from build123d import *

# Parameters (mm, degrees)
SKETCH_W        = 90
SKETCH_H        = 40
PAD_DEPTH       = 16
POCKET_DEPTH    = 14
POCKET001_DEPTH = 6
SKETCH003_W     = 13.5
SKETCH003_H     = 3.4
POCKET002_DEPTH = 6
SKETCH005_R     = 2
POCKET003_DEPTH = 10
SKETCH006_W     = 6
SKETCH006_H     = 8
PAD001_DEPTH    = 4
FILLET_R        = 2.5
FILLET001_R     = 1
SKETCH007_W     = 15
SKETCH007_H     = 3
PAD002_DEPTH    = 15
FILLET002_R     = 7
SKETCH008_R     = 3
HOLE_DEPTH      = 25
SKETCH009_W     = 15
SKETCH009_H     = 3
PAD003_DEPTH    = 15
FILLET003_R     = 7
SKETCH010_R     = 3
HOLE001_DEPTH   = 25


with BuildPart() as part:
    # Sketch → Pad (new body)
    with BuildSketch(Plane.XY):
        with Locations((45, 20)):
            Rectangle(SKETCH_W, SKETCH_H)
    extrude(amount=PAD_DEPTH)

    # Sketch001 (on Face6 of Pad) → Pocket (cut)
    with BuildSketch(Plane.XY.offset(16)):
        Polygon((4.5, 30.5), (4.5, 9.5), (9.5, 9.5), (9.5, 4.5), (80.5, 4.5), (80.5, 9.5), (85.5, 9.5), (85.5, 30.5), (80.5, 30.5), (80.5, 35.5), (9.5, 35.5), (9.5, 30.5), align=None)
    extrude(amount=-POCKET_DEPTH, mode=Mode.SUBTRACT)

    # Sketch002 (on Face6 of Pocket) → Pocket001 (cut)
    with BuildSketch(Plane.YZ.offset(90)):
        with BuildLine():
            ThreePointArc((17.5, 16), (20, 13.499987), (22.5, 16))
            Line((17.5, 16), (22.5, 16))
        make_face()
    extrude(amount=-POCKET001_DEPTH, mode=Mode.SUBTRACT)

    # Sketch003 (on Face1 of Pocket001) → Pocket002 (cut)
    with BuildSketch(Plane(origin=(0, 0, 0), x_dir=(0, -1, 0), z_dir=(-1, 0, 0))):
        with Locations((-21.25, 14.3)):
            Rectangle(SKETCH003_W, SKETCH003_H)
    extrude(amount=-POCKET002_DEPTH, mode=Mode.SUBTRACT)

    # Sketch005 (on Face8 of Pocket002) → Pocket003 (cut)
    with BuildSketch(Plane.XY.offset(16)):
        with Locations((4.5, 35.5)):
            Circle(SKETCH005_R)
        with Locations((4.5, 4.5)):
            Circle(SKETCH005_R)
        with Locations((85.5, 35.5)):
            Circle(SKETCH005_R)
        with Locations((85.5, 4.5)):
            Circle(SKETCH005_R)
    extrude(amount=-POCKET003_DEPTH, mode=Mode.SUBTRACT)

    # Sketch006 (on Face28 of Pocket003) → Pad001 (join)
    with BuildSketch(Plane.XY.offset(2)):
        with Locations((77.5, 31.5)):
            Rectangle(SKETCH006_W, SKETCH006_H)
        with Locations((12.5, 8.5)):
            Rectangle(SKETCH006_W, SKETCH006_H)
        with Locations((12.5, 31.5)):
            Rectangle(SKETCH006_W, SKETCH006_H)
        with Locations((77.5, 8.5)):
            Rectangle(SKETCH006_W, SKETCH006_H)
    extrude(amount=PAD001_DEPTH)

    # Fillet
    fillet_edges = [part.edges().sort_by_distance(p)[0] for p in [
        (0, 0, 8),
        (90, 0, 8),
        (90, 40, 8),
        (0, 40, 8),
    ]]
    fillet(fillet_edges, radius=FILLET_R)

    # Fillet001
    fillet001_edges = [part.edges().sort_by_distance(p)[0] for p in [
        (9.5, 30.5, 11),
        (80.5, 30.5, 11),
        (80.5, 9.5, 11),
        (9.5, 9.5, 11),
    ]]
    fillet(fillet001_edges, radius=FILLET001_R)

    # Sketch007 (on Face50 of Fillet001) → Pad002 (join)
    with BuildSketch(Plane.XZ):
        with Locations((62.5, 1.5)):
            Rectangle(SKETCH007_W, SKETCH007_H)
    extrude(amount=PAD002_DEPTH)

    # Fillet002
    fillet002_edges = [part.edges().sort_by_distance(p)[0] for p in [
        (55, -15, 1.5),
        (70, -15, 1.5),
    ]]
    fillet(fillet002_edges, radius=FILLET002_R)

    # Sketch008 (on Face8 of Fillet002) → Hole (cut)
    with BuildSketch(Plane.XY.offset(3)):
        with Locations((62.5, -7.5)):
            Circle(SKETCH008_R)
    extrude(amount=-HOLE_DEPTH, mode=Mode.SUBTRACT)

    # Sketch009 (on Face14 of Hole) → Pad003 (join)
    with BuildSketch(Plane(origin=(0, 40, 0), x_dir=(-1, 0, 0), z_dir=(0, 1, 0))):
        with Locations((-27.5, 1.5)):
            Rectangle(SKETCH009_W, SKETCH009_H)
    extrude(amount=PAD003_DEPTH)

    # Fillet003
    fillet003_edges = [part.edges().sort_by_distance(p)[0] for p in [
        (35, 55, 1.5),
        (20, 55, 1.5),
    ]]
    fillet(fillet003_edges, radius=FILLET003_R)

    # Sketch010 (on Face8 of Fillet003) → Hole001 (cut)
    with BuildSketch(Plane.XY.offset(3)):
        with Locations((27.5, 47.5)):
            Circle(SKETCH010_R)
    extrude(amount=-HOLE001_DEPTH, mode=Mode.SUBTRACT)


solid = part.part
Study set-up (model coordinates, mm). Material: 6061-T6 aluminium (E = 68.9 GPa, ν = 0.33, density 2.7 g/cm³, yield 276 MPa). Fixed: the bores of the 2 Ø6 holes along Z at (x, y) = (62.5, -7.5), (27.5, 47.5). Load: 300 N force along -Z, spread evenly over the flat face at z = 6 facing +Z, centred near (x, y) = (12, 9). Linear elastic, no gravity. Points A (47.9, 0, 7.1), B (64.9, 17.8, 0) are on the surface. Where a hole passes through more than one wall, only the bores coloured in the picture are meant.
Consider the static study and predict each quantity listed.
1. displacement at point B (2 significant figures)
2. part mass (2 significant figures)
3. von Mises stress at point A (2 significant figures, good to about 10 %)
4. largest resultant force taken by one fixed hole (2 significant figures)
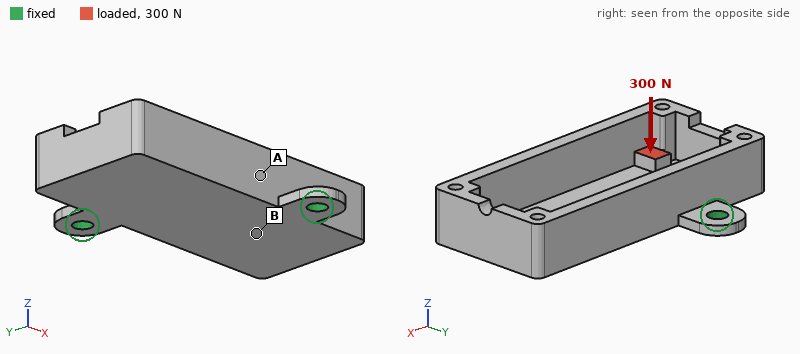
0.089 mm
67 g
23 MPa
170 N
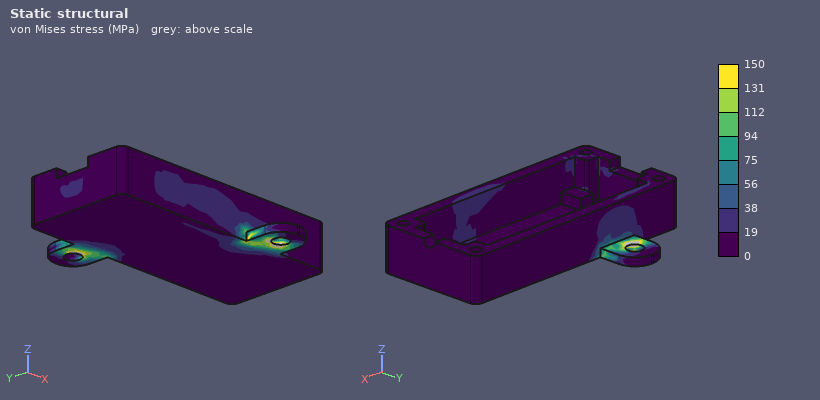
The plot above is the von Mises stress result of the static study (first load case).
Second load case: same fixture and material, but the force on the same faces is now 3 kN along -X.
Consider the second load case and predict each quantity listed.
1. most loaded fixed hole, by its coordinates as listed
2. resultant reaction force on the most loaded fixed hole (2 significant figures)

(62.5, -7.5)
2.0 kN
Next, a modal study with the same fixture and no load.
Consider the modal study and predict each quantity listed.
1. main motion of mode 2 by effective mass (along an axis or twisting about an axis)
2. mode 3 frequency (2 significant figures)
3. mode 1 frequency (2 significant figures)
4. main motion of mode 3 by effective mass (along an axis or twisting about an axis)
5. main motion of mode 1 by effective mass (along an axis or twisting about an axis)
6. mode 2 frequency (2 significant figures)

along Z
5000 Hz
840 Hz
along Z
twisting about Y
2100 Hz
